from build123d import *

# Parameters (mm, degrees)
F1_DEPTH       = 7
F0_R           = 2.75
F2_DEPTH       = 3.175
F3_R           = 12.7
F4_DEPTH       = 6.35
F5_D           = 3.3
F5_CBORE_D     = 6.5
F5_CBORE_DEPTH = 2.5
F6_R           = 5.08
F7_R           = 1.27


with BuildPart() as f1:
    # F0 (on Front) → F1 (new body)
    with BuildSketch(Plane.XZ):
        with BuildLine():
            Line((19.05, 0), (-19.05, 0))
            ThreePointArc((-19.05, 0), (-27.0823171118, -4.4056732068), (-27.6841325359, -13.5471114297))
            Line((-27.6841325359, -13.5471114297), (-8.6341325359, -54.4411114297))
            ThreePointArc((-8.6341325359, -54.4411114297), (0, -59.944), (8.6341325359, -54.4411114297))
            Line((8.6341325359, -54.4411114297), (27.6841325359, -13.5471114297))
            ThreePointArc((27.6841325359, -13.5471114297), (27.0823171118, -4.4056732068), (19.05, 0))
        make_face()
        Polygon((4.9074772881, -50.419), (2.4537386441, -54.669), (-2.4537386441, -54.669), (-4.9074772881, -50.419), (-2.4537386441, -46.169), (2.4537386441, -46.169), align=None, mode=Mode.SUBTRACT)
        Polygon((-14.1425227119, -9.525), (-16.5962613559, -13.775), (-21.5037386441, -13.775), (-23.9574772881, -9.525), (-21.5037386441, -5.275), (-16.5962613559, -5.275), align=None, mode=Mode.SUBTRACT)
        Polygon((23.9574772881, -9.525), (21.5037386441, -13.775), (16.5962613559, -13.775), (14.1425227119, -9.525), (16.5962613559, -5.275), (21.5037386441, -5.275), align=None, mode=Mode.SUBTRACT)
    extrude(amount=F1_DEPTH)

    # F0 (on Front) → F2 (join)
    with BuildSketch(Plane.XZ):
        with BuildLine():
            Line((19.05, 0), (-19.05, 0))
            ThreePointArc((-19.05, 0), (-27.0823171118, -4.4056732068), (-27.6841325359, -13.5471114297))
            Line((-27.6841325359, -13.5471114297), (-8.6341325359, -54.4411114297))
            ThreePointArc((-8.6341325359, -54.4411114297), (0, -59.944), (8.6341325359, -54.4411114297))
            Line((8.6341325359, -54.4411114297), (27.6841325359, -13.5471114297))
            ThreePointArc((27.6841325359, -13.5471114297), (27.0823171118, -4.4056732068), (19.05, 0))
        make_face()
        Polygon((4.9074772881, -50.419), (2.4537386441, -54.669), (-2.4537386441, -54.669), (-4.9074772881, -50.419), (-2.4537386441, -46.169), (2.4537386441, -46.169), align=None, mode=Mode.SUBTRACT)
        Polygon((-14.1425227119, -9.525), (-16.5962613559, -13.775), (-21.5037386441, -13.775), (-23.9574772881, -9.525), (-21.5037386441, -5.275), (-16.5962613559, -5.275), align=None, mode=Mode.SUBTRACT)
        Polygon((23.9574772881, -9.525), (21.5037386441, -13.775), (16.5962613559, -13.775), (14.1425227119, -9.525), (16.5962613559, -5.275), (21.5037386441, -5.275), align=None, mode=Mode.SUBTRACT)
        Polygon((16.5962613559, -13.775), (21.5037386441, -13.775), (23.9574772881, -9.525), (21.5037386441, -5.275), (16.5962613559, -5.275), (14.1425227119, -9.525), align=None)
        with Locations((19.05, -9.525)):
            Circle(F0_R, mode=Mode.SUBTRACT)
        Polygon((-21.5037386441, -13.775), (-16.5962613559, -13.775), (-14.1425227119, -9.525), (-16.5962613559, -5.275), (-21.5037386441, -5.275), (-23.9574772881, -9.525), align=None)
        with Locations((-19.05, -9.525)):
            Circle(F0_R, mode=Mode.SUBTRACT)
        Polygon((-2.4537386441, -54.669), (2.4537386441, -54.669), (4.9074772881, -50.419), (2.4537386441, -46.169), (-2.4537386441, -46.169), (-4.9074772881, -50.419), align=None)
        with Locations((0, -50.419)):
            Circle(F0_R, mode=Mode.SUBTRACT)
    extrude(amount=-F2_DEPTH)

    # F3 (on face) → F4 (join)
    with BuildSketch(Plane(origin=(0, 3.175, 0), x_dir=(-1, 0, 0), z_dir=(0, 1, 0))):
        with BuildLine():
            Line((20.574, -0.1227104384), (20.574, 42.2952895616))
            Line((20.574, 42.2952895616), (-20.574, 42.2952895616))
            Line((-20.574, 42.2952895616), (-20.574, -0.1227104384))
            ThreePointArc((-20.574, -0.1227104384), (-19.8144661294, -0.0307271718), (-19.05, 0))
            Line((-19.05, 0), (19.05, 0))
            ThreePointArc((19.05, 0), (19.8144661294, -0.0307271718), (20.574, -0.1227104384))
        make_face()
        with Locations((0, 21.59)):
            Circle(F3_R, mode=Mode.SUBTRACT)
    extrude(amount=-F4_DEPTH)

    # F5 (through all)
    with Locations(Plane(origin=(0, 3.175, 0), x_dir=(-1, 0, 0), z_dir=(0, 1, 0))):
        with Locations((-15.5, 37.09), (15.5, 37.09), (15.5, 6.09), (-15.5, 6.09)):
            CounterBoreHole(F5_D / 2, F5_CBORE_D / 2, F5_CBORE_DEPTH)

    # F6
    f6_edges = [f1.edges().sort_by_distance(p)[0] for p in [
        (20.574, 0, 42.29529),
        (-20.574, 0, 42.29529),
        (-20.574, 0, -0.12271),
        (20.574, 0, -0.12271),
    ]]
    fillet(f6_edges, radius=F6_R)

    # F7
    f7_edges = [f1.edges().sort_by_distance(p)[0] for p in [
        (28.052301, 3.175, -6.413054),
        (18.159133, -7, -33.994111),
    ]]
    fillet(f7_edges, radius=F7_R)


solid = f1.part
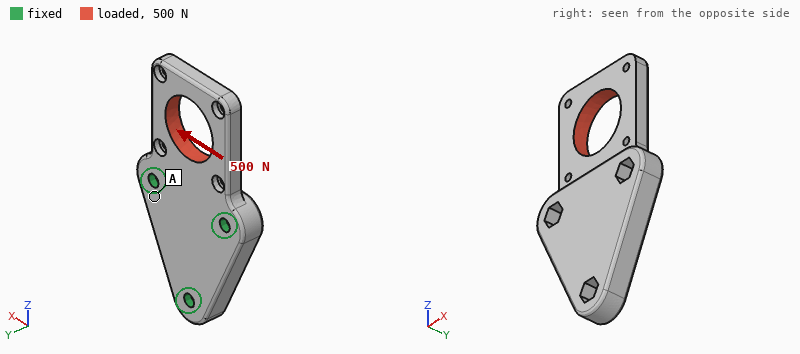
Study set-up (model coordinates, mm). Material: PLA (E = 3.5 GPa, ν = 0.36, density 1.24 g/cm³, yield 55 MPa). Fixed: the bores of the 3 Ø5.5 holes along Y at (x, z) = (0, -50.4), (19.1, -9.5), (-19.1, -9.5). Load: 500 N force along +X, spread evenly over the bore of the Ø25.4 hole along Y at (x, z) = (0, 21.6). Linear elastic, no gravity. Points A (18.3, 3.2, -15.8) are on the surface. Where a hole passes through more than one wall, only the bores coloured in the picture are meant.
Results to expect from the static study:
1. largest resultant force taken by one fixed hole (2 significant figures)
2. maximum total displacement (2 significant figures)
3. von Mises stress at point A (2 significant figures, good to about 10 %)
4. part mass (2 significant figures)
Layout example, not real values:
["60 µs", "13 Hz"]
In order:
["430 N", "0.32 mm", "2.8 MPa", "36 g"]
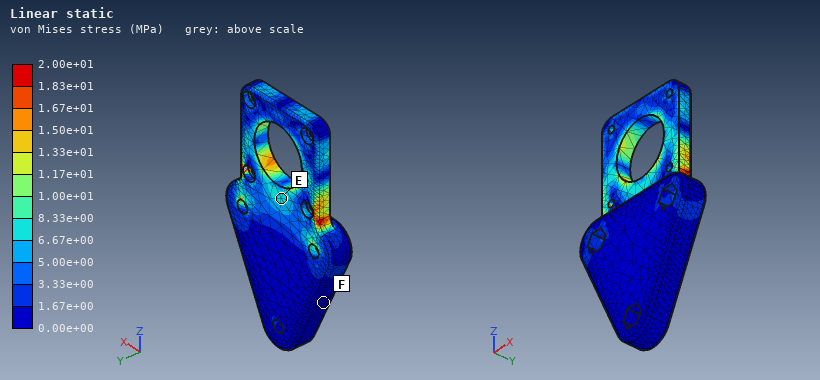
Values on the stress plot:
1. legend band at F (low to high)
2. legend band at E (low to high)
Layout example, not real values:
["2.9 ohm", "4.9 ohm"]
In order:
["0.00e+00 to 1.67e+00 MPa", "6.67e+00 to 8.33e+00 MPa"]
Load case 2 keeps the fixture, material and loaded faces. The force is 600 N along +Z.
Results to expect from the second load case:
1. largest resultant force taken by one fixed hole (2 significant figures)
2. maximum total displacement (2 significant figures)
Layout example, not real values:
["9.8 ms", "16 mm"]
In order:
["250 N", "93 µm"]
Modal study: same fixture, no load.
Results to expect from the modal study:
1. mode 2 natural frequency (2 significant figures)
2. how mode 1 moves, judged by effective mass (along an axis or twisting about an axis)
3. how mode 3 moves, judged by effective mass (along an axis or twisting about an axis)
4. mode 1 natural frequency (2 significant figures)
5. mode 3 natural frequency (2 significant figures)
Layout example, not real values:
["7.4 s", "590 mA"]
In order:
["1600 Hz", "along Y", "along X", "680 Hz", "2400 Hz"]
